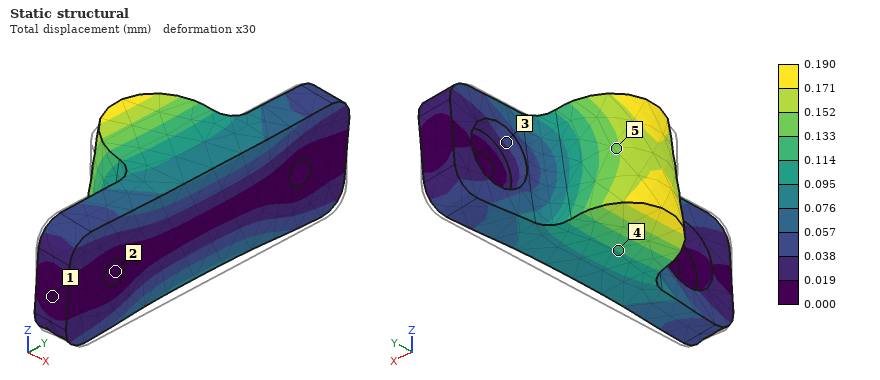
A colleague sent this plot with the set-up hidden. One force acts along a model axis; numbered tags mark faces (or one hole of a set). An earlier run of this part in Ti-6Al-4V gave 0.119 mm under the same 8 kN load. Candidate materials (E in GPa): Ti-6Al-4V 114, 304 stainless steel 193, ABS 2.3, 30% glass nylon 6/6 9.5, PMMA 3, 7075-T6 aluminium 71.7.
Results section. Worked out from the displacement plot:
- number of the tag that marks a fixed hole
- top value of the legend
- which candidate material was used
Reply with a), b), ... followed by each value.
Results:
a) 2
b) 0.190 mm
c) 7075-T6 aluminium
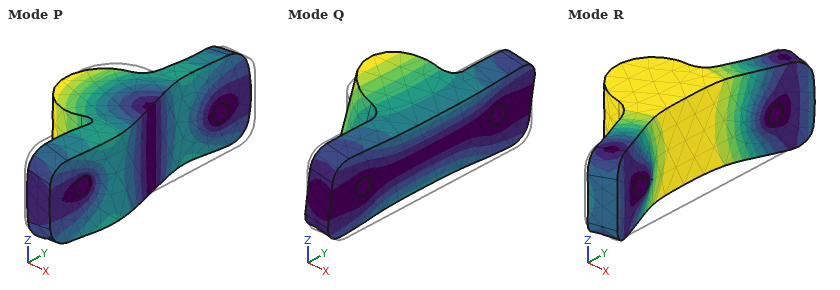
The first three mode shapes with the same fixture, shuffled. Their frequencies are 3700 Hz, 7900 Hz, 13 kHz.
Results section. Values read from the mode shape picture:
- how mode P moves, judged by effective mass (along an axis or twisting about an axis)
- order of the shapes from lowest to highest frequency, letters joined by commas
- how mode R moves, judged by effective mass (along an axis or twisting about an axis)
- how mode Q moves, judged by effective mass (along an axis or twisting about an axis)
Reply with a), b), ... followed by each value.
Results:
a) along Y
b) Q, R, P
c) along X
d) along Z
